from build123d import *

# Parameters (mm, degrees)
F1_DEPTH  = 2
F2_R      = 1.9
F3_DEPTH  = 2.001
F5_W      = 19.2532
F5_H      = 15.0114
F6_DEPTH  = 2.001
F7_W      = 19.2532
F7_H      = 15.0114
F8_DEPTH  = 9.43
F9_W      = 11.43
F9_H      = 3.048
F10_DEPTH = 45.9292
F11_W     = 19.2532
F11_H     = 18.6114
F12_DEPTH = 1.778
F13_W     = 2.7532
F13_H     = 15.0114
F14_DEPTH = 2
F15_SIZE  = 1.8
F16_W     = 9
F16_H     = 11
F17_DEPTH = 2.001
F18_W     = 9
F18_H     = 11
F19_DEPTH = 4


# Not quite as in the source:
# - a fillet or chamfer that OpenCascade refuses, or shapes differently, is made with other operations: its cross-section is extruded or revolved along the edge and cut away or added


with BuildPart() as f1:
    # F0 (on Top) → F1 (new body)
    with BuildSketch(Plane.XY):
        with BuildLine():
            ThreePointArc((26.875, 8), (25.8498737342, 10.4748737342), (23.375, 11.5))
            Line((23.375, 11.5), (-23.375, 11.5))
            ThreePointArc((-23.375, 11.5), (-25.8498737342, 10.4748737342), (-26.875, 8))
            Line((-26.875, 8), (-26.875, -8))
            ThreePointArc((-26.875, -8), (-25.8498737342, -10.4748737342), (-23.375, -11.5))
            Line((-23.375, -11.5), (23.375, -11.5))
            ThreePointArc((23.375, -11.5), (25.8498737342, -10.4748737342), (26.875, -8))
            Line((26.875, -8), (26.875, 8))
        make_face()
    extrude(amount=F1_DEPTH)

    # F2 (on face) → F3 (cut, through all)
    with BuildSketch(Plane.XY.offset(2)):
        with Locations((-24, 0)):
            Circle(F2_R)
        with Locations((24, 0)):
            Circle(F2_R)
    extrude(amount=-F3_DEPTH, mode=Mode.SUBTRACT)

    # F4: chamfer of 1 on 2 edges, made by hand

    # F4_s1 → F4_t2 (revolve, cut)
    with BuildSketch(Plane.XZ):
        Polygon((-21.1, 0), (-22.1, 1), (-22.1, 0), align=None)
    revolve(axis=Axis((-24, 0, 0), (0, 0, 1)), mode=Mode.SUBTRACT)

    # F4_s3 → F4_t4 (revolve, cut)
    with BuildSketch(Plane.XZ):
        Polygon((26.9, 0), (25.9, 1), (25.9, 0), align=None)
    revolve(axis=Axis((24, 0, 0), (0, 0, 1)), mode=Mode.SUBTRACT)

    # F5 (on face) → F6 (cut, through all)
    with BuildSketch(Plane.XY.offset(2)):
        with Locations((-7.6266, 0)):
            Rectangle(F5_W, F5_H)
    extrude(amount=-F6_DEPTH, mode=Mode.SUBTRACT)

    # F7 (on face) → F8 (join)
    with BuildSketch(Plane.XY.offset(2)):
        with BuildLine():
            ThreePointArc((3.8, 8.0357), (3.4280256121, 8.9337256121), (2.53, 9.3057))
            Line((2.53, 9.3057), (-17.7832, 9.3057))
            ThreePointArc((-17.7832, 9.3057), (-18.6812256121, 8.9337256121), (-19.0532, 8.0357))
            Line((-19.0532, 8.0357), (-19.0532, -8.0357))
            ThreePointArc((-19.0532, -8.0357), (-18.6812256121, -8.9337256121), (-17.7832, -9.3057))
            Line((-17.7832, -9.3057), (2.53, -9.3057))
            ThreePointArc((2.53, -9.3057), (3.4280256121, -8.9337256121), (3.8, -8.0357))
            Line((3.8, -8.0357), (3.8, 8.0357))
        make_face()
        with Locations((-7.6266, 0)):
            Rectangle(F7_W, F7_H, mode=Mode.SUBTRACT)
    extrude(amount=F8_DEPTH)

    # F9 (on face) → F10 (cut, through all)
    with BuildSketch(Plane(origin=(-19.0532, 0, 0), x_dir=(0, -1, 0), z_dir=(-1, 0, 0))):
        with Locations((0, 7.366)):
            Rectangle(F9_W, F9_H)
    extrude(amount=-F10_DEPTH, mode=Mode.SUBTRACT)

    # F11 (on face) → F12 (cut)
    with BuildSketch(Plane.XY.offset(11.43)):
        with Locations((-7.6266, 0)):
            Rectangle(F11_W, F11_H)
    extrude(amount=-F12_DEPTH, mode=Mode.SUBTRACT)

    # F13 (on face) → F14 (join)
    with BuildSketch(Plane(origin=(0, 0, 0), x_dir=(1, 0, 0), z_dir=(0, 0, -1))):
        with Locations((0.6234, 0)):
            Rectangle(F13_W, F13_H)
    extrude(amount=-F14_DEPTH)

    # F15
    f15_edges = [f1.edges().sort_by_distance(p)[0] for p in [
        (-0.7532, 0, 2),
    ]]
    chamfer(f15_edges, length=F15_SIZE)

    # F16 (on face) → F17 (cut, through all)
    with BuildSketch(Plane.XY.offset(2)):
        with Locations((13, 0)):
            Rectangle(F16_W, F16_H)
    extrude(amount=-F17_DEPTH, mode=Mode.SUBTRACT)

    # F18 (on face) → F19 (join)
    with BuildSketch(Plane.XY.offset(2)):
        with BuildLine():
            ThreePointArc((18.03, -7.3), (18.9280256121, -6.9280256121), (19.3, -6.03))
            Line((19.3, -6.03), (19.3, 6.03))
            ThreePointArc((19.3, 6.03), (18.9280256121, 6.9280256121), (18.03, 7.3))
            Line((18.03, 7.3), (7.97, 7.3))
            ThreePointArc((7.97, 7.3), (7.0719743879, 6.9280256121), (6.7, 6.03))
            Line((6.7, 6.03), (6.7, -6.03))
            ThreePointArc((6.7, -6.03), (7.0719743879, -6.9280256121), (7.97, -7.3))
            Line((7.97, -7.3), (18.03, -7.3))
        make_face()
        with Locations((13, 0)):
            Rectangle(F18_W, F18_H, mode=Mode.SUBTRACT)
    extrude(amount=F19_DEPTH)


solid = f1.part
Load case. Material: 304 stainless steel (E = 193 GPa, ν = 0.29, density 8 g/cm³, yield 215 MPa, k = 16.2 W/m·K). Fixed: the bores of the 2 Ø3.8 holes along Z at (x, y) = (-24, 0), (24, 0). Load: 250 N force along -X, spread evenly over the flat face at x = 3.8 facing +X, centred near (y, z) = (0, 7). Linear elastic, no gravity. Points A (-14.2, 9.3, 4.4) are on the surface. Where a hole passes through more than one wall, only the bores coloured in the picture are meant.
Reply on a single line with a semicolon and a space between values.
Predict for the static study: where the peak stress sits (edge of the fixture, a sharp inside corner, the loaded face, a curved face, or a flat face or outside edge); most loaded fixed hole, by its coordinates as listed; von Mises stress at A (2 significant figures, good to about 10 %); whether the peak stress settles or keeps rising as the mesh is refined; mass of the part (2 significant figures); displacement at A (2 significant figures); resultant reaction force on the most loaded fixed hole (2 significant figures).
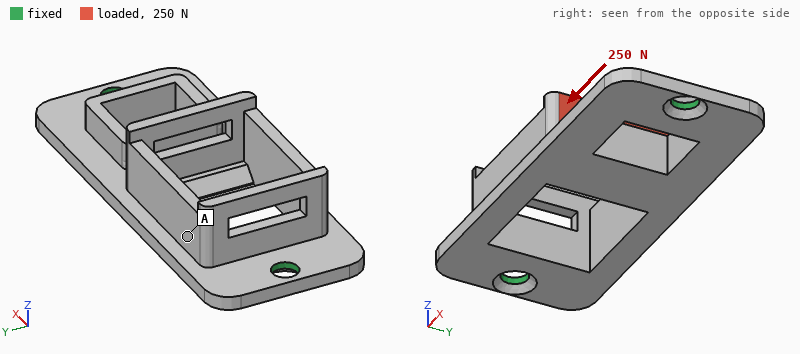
edge of the fixture; (24, 0); 7.1 MPa; keeps rising; 24 g; 2.4 µm; 140 N
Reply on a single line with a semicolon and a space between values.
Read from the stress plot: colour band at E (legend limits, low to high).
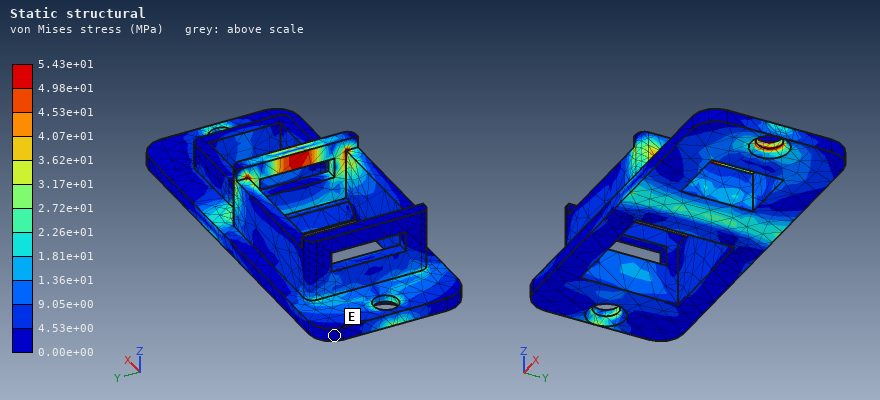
0.00e+00 to 4.53e+00 MPa
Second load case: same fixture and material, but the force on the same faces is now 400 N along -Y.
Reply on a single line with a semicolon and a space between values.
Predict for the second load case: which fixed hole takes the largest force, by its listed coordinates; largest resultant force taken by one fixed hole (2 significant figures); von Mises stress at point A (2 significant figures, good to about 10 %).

(24, 0); 270 N; 26 MPa
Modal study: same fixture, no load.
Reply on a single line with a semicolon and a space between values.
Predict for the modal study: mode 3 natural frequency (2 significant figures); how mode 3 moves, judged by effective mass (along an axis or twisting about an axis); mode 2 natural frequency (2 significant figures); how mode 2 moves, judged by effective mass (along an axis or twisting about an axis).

8700 Hz; along Y; 3800 Hz; along Z
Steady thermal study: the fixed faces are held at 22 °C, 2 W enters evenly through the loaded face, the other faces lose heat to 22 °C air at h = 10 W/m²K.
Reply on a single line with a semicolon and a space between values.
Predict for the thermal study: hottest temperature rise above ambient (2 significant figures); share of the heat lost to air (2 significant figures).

58 K; 34 %
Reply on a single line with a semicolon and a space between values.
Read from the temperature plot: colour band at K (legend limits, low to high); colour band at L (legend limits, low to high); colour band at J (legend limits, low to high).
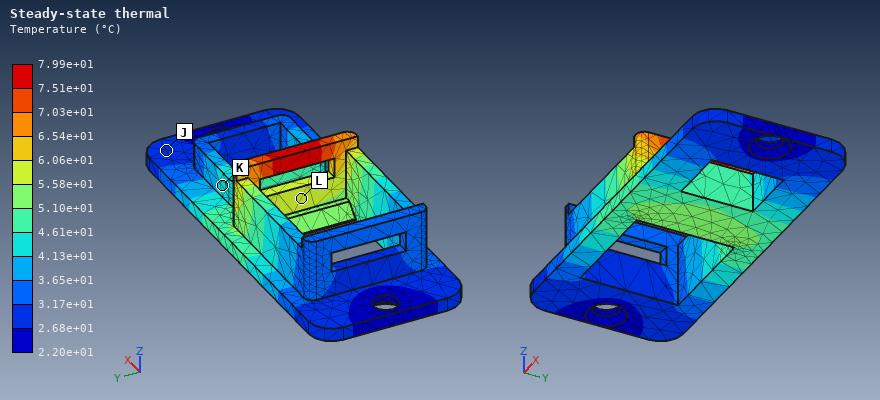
4.13e+01 to 4.61e+01 °C; 5.58e+01 to 6.06e+01 °C; 2.68e+01 to 3.17e+01 °C
